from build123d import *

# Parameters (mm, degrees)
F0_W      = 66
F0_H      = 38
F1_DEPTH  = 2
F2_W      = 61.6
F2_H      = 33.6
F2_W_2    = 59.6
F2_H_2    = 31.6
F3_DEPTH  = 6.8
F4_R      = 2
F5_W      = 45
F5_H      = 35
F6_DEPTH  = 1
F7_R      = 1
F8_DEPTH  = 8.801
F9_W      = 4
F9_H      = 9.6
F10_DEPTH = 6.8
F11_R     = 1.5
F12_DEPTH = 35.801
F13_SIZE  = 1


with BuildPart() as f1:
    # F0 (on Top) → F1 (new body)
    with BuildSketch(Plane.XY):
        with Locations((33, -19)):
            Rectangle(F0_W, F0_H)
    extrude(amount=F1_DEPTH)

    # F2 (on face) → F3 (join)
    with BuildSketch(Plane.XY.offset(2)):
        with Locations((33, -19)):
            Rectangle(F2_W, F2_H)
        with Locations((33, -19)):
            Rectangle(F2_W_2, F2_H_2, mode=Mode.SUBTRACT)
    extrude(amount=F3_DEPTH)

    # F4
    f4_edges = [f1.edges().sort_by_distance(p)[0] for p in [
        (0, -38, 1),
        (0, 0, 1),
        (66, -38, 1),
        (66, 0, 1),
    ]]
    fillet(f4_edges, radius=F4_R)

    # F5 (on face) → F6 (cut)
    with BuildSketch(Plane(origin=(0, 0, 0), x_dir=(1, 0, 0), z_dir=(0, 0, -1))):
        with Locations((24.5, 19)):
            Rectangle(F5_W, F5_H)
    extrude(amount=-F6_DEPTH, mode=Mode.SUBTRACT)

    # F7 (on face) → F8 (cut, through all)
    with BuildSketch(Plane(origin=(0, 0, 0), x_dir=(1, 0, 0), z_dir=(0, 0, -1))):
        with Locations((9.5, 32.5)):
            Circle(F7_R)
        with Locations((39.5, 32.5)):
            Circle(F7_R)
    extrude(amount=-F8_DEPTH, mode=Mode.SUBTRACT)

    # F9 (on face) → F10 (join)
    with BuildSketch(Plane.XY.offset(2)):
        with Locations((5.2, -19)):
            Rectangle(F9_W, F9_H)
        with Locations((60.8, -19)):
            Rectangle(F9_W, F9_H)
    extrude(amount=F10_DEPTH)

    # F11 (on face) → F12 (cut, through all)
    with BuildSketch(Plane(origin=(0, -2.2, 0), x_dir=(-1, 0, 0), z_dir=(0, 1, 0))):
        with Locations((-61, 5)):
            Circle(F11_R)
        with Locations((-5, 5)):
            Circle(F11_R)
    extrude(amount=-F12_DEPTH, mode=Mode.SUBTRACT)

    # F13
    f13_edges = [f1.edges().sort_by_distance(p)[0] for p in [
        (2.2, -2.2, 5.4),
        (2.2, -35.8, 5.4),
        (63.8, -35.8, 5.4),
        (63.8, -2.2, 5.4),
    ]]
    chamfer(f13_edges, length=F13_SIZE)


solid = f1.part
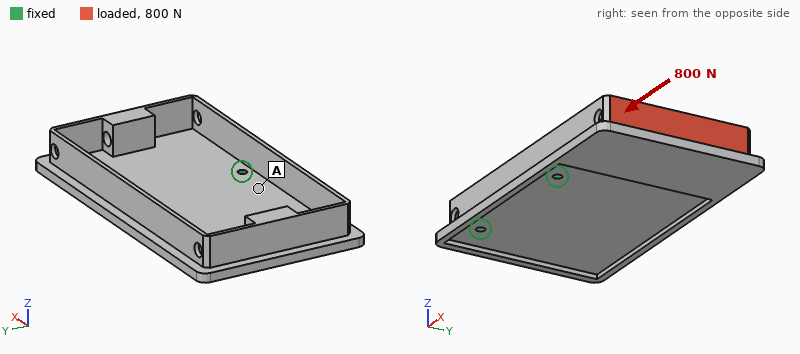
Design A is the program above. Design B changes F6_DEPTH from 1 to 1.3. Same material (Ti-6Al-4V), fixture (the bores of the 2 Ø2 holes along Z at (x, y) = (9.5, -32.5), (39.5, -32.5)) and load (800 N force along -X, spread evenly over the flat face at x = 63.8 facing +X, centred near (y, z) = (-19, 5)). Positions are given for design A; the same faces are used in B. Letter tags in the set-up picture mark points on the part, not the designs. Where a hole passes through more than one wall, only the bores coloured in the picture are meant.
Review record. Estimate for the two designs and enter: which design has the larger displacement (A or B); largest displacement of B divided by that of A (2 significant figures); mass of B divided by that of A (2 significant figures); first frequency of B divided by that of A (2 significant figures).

B
1.2
0.91
0.72
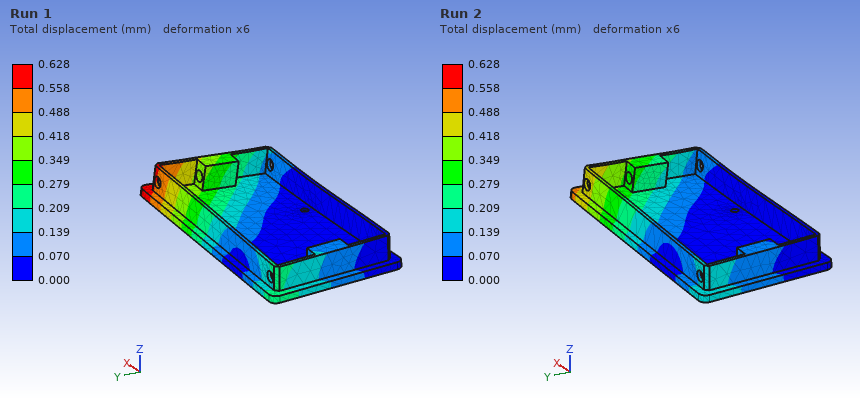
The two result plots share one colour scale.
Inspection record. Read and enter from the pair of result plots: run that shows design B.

Run 1
